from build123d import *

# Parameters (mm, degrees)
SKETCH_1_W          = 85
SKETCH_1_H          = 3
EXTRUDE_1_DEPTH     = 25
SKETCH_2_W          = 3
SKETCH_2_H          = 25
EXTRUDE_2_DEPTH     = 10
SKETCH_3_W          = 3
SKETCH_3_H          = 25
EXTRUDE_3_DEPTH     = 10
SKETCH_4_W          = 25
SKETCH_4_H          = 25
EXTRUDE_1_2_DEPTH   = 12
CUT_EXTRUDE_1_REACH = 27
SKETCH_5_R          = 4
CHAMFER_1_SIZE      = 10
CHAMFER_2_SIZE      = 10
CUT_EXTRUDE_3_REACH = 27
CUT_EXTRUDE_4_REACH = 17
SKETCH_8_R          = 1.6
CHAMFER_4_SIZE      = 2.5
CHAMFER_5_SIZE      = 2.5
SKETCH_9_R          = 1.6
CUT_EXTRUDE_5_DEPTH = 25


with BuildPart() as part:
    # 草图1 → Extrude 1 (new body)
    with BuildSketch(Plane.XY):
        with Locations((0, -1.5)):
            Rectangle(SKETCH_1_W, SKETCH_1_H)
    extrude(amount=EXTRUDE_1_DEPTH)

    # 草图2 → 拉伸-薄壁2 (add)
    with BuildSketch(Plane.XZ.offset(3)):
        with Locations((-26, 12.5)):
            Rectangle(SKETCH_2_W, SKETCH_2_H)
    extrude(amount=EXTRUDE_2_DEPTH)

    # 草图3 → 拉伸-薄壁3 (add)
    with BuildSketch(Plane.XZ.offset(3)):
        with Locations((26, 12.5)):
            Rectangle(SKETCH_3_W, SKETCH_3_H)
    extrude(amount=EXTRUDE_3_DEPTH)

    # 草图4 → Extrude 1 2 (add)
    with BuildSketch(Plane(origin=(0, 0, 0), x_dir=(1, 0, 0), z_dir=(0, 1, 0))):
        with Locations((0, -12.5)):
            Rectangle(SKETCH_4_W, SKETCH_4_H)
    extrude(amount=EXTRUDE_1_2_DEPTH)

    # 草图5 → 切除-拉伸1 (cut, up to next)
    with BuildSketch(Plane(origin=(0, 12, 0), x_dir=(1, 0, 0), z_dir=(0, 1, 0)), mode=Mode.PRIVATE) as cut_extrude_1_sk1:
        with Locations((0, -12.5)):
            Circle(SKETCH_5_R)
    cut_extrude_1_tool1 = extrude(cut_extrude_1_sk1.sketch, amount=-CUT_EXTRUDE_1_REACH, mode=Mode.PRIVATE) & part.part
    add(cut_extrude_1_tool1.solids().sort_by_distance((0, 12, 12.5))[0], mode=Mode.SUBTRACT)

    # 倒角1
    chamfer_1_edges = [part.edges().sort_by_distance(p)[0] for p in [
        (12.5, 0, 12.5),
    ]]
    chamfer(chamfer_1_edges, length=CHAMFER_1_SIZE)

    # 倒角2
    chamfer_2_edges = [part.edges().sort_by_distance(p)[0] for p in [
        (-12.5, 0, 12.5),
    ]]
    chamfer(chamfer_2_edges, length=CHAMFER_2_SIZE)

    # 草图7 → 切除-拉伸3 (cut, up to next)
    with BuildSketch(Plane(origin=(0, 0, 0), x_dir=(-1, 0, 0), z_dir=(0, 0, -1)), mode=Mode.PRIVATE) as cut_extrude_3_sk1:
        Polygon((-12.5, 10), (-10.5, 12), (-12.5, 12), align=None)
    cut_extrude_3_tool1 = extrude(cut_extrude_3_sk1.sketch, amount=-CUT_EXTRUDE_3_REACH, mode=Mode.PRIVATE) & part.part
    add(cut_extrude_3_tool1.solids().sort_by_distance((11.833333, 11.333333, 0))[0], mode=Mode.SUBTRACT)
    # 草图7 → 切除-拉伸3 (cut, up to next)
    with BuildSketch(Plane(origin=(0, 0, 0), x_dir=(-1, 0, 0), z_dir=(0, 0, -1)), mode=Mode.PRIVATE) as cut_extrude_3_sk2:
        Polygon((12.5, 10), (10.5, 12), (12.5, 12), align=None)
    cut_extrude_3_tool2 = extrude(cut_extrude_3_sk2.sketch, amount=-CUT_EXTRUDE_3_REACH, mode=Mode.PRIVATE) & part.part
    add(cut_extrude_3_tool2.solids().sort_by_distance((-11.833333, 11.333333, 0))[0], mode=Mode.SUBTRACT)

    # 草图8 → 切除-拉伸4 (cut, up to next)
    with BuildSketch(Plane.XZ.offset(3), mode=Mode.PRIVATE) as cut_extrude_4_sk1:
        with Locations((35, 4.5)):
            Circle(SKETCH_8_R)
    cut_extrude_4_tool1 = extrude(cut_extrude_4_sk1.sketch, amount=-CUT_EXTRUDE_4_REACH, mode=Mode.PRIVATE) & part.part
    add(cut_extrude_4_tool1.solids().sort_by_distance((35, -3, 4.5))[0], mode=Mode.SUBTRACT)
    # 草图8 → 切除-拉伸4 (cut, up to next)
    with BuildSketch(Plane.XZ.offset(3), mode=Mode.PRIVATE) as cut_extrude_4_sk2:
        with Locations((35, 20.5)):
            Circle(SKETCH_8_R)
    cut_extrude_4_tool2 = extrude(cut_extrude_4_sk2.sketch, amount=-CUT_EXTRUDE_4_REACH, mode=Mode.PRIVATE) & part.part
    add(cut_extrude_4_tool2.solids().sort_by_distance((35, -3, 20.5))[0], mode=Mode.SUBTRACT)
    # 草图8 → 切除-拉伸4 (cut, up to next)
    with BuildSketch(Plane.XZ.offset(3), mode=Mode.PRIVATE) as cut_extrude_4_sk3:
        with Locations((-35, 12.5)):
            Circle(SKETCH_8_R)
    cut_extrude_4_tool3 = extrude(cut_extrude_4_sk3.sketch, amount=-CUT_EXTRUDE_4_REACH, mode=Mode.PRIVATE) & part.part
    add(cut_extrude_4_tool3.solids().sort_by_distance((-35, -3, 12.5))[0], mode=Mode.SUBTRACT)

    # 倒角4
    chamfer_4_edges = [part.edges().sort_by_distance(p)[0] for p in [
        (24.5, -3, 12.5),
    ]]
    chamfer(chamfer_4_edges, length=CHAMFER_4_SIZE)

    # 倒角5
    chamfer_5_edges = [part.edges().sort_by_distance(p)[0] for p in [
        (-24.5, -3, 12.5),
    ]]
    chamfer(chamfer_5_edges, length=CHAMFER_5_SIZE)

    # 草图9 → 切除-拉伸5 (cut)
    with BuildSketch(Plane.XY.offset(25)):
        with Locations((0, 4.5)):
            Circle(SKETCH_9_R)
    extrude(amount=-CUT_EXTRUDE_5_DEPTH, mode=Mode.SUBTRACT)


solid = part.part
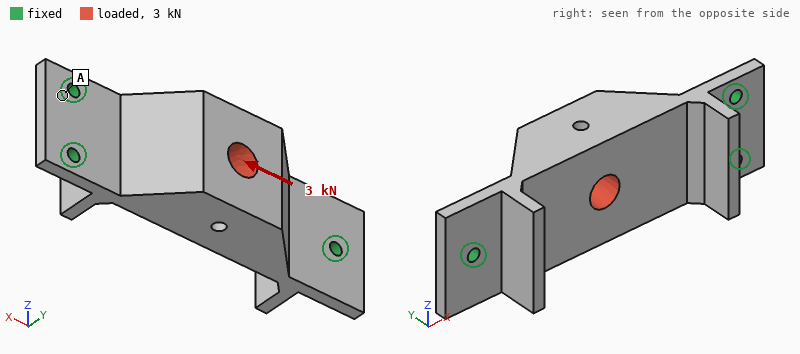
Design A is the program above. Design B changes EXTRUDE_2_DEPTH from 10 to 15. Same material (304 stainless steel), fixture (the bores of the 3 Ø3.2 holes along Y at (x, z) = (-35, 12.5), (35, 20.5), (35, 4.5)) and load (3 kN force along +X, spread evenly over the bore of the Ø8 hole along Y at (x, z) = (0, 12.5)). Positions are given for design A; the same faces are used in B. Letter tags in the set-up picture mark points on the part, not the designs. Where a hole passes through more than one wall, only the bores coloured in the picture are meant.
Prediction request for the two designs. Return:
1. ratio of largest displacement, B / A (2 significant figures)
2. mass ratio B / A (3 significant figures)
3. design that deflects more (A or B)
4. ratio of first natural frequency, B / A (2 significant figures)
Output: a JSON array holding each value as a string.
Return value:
["1.1", "1.02", "B", "0.98"]
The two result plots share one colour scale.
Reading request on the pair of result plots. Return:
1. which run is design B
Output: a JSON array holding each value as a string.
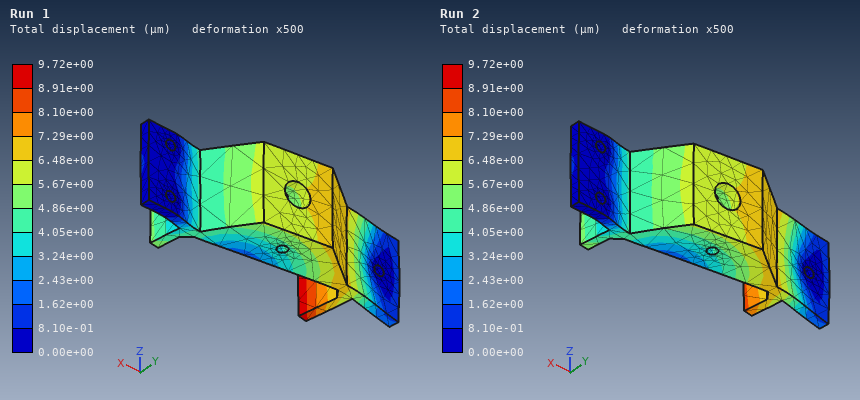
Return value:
["Run 1"]
